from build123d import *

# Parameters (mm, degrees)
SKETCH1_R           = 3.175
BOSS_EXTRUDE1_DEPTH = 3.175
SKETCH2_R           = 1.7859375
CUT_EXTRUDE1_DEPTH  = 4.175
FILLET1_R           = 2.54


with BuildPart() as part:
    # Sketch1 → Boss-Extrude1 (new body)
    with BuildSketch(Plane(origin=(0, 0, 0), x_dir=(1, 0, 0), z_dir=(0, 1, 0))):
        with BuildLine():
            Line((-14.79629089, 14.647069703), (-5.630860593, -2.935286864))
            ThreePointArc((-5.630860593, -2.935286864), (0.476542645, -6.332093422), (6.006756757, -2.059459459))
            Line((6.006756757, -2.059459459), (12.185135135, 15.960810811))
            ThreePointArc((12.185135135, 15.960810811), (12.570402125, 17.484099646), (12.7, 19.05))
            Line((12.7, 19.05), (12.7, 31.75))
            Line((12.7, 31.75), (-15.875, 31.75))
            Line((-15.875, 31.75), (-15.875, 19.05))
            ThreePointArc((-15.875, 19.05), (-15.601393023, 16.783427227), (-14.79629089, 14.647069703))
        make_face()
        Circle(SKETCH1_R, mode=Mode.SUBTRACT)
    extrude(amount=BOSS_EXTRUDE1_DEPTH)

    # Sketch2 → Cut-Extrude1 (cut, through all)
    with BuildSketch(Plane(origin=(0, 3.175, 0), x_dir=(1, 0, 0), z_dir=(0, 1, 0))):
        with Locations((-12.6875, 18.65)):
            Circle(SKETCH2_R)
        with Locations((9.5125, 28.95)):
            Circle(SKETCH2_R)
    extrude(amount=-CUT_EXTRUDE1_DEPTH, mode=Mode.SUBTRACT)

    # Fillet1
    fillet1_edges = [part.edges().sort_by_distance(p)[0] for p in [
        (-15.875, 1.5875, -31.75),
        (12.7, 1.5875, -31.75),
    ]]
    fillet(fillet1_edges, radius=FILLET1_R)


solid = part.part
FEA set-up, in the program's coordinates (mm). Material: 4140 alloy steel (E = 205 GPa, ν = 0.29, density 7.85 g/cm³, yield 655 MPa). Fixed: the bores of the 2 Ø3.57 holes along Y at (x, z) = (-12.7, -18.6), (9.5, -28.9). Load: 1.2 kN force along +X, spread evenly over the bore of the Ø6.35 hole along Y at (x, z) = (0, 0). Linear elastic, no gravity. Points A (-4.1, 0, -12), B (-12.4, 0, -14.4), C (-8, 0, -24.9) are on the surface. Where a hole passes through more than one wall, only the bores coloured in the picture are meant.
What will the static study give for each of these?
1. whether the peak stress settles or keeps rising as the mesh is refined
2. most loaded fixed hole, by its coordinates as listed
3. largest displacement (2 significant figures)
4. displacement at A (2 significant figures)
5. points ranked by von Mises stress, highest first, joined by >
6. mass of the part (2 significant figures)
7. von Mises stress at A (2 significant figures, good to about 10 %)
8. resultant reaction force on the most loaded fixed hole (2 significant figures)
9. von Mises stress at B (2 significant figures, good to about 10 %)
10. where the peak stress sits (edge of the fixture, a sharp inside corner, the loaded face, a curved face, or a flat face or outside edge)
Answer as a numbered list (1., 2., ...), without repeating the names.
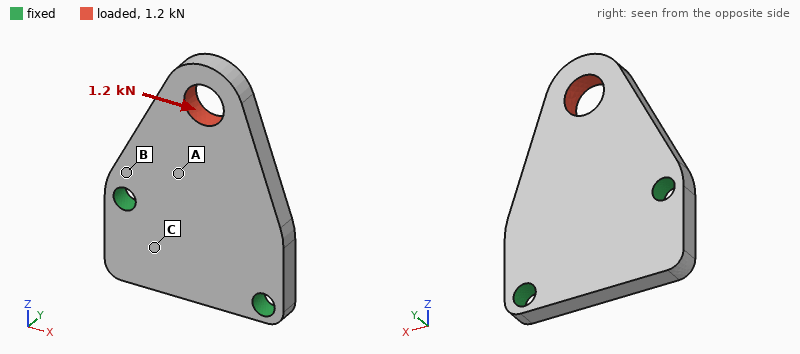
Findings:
1. keeps rising
2. (-12.7, -18.6)
3. 15 µm
4. 2.5 µm
5. B > A > C
6. 20 g
7. 30 MPa
8. 1.5 kN
9. 61 MPa
10. edge of the fixture
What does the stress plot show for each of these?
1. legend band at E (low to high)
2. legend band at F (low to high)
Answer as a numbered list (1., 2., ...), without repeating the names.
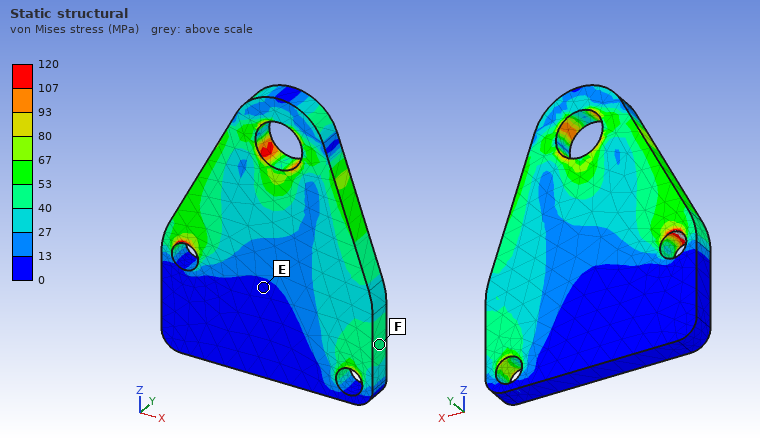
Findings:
1. 0 to 13 MPa
2. 40 to 53 MPa
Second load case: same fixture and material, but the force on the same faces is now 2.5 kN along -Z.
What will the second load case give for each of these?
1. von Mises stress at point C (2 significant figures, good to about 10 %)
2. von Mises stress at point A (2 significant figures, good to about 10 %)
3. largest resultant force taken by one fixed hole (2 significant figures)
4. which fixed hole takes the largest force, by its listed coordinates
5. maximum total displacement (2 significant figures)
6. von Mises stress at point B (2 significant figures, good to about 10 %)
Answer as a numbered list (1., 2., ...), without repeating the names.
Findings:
1. 16 MPa
2. 29 MPa
3. 1.5 kN
4. (9.5, -28.9)
5. 9.4 µm
6. 32 MPa
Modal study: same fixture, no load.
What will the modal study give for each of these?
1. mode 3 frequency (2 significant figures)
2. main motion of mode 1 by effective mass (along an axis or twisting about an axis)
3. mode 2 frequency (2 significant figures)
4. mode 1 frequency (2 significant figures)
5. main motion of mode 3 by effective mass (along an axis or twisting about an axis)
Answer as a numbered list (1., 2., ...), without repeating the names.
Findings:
1. 19 kHz
2. along Y
3. 14 kHz
4. 4600 Hz
5. along Y
